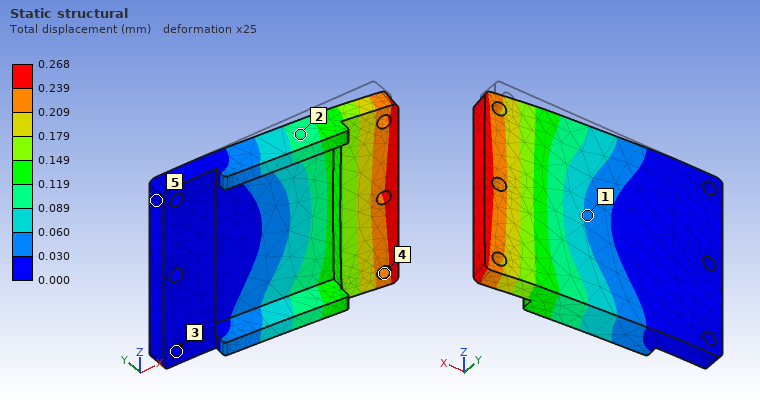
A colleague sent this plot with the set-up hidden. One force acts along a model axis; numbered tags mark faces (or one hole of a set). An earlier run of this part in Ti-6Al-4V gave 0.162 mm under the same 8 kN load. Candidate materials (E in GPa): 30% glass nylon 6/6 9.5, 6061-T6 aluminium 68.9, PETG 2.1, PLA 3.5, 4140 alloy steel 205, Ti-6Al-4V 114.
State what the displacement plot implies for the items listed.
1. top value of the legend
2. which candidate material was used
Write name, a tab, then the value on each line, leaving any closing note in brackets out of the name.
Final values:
top value of the legend	0.268 mm
which candidate material was used	6061-T6 aluminium
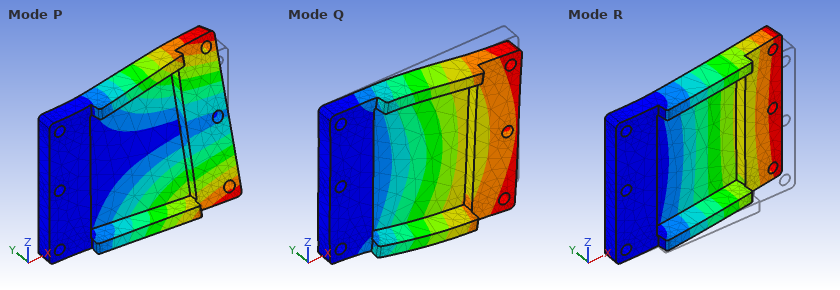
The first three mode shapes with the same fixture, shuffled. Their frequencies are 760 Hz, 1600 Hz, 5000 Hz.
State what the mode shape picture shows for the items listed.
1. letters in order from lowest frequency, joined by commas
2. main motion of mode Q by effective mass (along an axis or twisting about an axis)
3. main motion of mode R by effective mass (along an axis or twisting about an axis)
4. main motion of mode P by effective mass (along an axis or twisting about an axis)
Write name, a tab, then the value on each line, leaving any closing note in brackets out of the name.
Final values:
letters in order from lowest frequency, joined by commas	R, P, Q
main motion of mode Q by effective mass	along Z
main motion of mode R by effective mass	along Y
main motion of mode P by effective mass	twisting about X
